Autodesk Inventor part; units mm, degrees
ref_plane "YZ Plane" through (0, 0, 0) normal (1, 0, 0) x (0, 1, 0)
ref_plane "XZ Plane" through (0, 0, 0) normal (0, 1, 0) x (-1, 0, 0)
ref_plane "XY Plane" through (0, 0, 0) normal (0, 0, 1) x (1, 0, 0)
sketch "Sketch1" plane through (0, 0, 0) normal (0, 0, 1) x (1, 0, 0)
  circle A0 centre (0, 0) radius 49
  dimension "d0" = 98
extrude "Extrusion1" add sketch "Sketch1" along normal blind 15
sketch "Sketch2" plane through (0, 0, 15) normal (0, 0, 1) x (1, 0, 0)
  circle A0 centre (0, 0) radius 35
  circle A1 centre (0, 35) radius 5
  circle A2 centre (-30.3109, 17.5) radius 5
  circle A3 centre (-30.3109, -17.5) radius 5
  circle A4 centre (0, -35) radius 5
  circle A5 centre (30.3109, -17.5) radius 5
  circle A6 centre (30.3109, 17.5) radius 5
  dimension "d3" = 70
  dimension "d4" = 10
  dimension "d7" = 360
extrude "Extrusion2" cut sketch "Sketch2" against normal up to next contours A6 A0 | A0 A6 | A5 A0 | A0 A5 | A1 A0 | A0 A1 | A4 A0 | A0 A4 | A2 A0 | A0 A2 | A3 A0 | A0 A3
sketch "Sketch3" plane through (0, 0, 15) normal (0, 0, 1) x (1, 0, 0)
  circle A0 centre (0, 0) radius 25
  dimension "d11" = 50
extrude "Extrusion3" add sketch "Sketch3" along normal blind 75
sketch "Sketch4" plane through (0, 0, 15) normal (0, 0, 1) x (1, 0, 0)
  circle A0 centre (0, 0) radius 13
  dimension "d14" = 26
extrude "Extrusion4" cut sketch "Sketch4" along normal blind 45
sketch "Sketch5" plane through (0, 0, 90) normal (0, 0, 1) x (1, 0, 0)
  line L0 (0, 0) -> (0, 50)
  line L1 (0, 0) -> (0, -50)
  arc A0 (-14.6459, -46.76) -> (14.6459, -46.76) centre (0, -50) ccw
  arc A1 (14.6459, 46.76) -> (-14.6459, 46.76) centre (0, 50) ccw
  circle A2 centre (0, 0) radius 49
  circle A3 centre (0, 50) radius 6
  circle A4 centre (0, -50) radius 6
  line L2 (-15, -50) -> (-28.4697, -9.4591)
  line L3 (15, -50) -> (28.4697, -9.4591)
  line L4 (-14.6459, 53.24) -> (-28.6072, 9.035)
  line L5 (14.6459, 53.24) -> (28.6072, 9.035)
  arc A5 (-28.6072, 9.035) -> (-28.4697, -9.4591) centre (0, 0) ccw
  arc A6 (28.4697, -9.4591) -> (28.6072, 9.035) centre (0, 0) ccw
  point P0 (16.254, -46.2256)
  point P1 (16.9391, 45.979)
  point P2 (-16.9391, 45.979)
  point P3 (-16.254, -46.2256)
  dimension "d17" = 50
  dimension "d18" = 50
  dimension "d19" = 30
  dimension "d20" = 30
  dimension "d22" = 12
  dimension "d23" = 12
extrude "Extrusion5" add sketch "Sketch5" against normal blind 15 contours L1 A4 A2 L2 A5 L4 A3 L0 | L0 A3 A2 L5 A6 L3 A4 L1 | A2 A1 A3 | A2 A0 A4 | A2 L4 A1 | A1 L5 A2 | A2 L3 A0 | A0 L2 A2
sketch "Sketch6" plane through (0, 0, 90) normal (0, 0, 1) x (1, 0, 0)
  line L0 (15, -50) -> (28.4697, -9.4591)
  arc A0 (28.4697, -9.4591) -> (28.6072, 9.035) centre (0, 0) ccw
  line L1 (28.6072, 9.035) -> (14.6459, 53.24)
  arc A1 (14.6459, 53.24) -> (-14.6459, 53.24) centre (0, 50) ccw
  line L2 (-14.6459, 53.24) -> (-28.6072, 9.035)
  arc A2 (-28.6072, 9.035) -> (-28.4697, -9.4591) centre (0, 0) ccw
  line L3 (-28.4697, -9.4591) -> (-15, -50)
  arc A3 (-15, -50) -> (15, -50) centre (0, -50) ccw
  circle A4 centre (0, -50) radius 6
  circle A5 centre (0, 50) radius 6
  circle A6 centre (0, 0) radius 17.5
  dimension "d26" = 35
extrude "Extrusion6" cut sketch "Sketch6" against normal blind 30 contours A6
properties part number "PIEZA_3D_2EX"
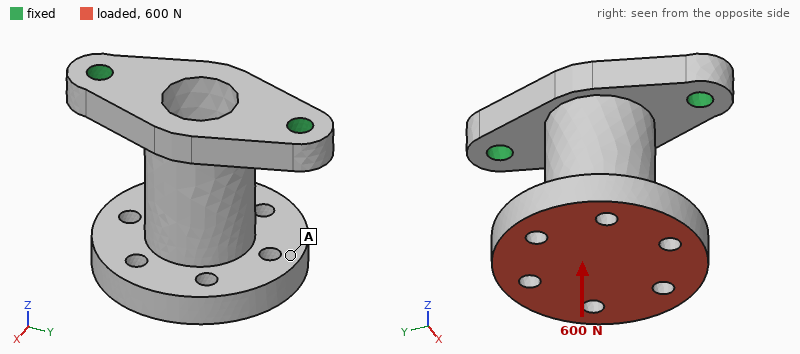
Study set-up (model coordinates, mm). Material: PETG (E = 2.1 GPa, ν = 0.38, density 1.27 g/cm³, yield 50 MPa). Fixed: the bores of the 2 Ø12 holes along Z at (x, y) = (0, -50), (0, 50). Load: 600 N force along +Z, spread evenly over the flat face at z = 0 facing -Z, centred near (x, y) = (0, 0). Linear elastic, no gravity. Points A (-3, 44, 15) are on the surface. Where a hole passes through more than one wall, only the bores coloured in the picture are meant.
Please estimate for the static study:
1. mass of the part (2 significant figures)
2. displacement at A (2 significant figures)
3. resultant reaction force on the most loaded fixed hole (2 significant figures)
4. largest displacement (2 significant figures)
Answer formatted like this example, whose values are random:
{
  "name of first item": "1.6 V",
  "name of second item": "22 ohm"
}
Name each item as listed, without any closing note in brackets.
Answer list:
{
  "mass of the part": "320 g",
  "displacement at A": "0.098 mm",
  "resultant reaction force on the most loaded fixed hole": "320 N",
  "largest displacement": "0.10 mm"
}
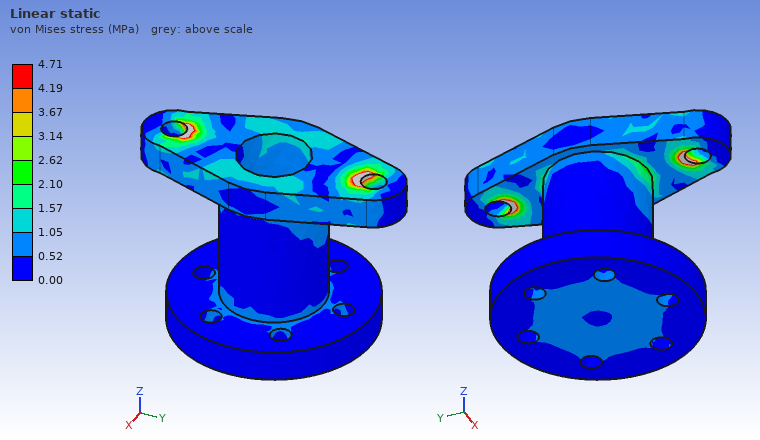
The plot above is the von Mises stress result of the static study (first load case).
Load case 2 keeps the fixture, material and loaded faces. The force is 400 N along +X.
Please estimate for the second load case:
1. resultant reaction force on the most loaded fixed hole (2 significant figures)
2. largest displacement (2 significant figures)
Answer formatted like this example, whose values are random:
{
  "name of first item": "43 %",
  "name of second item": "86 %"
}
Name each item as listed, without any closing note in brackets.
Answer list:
{
  "resultant reaction force on the most loaded fixed hole": "200 N",
  "largest displacement": "1.8 mm"
}
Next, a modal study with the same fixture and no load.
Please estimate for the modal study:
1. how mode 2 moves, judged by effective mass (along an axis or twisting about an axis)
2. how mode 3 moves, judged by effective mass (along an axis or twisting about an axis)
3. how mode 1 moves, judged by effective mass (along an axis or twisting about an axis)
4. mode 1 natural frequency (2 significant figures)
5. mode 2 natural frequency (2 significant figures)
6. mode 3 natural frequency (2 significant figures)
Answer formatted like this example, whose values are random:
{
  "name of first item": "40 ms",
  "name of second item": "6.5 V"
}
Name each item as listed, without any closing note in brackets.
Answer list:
{
  "how mode 2 moves, judged by effective mass": "along Y",
  "how mode 3 moves, judged by effective mass": "along Z",
  "how mode 1 moves, judged by effective mass": "along X",
  "mode 1 natural frequency": "210 Hz",
  "mode 2 natural frequency": "430 Hz",
  "mode 3 natural frequency": "840 Hz"
}
